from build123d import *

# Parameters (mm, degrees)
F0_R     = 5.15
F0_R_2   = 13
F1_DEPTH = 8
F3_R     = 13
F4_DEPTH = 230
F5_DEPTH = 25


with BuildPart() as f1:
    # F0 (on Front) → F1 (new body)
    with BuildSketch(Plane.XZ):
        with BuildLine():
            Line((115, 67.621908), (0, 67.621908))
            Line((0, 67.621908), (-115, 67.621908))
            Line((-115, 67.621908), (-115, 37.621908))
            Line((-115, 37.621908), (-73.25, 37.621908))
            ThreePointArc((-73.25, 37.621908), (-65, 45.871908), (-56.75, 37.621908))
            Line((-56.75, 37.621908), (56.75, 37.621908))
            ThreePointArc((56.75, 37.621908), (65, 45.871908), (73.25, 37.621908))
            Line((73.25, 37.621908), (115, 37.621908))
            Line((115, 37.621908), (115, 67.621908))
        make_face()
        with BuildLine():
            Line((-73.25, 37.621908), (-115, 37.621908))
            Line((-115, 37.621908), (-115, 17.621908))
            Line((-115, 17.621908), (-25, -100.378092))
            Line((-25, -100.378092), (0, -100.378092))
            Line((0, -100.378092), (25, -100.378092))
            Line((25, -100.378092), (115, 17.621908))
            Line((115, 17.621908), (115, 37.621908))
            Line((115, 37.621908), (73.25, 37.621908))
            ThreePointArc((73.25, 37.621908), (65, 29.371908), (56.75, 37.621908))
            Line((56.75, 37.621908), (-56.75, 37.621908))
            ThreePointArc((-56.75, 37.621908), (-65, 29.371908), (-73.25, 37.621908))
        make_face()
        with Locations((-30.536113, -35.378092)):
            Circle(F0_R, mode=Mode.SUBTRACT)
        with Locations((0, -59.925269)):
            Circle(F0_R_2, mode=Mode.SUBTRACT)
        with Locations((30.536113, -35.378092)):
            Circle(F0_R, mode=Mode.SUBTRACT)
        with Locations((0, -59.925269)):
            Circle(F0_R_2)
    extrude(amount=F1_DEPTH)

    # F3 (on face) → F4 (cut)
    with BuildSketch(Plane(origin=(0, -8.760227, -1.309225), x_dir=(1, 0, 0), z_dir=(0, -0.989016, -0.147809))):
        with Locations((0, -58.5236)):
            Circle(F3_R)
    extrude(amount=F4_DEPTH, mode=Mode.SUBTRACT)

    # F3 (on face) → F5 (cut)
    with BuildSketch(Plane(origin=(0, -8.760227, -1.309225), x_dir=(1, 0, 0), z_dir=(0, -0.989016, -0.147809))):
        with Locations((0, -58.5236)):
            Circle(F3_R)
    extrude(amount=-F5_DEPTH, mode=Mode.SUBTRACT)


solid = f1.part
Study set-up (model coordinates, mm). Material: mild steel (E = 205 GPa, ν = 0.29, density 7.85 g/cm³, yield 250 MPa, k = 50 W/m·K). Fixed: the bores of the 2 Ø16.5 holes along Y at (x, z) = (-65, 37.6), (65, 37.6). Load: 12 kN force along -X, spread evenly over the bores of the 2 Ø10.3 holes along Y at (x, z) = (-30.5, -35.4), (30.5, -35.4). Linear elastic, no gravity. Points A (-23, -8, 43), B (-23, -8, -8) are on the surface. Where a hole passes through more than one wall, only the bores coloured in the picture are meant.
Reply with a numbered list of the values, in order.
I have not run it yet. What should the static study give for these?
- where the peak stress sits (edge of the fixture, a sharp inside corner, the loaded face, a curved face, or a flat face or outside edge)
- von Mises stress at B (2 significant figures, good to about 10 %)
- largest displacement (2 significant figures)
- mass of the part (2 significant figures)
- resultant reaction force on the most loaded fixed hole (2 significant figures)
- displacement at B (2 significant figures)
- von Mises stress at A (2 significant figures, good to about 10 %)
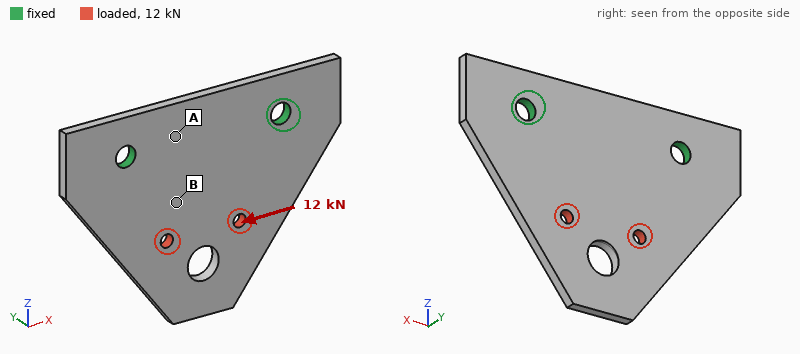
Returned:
1. edge of the fixture
2. 19 MPa
3. 13 µm
4. 1.7 kg
5. 8.6 kN
6. 6.9 µm
7. 7.0 MPa
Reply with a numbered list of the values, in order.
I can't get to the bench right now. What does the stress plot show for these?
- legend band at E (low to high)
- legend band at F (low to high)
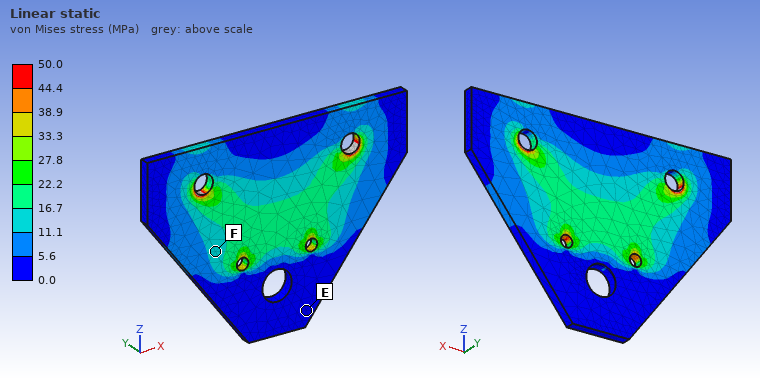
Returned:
1. 0.0 to 5.6 MPa
2. 11.1 to 16.7 MPa
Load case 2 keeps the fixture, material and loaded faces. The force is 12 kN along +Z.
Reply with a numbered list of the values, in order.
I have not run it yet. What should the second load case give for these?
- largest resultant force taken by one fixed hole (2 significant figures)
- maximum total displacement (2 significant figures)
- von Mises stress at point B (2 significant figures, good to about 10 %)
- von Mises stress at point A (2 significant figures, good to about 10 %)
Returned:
1. 6.3 kN
2. 7.0 µm
3. 9.6 MPa
4. 5.1 MPa
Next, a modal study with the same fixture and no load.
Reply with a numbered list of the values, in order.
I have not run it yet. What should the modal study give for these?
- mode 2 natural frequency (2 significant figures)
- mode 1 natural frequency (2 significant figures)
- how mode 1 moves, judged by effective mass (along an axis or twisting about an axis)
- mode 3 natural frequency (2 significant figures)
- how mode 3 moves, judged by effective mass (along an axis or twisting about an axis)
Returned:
1. 1400 Hz
2. 490 Hz
3. along Y
4. 2000 Hz
5. along Y
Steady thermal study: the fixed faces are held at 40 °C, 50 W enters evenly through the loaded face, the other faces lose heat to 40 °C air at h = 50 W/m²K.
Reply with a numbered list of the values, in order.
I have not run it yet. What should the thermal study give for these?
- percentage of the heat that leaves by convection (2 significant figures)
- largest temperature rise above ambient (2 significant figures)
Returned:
1. 70 %
2. 39 K
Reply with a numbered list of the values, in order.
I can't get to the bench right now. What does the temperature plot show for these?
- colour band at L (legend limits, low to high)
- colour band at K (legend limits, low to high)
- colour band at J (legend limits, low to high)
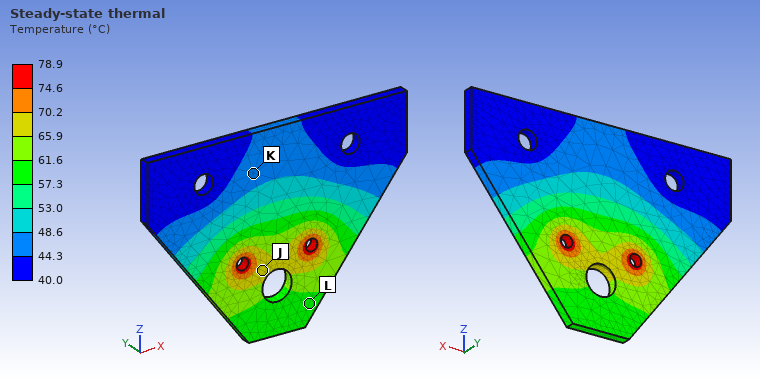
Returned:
1. 57.3 to 61.6 °C
2. 44.3 to 48.6 °C
3. 65.9 to 70.2 °C
